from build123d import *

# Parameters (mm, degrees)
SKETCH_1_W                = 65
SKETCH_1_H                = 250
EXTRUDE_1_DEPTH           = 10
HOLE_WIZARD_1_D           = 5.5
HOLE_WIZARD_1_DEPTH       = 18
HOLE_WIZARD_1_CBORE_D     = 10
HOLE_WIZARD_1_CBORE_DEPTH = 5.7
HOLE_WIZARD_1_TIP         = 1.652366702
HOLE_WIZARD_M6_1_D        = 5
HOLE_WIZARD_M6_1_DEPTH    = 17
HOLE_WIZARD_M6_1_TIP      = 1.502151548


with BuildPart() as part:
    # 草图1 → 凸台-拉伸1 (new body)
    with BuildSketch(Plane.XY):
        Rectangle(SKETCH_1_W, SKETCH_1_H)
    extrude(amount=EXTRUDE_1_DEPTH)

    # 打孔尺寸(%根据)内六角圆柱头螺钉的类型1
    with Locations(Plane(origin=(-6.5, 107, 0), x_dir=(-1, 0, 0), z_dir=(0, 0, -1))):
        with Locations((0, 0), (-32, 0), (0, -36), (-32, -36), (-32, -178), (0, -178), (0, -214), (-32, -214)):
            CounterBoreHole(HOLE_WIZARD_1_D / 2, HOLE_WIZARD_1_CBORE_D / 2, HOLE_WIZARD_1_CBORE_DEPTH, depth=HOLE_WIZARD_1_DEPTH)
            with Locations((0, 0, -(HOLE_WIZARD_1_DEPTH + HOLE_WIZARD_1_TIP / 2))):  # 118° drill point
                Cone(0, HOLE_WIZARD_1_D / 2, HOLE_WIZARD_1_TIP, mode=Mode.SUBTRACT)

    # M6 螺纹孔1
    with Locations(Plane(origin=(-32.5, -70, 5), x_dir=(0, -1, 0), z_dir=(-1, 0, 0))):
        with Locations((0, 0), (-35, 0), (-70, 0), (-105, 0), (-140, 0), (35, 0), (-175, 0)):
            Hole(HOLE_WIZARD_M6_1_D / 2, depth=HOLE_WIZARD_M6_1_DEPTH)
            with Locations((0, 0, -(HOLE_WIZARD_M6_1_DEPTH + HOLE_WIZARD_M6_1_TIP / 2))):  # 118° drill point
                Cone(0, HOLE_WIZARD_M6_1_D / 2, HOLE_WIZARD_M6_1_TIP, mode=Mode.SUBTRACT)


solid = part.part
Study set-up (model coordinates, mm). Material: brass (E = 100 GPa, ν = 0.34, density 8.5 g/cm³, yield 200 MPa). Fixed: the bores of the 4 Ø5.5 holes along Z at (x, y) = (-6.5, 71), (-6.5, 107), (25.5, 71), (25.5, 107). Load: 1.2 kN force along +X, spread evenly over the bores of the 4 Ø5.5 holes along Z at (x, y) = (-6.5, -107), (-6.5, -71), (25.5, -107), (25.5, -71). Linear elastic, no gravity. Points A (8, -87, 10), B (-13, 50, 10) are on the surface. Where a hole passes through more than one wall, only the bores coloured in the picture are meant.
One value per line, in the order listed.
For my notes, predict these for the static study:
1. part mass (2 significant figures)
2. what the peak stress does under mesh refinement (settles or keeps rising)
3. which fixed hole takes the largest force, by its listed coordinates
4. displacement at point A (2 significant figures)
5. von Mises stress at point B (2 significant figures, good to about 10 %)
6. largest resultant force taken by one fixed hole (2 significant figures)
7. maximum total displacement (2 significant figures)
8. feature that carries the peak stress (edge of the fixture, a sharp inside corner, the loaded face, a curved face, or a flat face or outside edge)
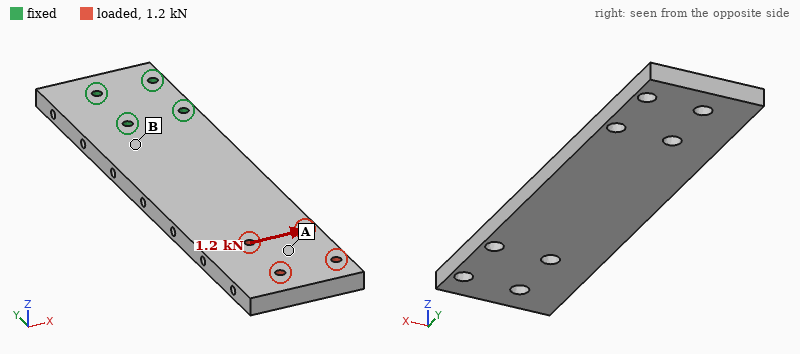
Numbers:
1.3 kg
keeps rising
(25.5, 71)
0.12 mm
14 MPa
3.6 kN
0.16 mm
edge of the fixture
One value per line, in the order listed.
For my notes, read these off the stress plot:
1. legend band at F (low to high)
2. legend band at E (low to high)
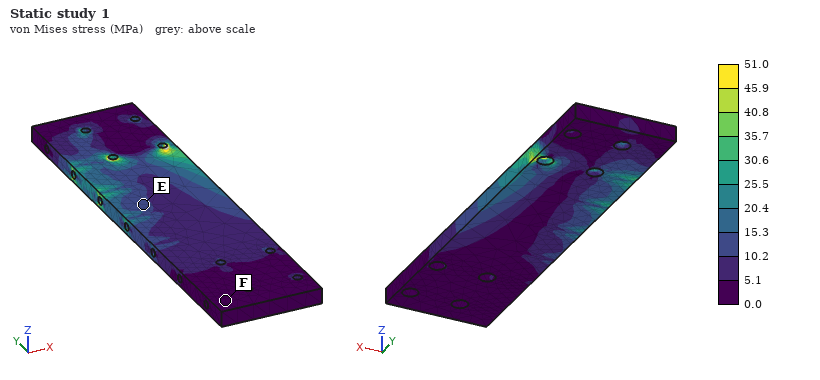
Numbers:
0.0 to 5.1 MPa
10.2 to 15.3 MPa
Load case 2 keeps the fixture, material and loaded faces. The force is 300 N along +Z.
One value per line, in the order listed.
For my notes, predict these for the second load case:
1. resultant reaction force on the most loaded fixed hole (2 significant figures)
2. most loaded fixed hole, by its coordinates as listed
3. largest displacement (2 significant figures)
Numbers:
1.6 kN
(-6.5, 71)
1.2 mm
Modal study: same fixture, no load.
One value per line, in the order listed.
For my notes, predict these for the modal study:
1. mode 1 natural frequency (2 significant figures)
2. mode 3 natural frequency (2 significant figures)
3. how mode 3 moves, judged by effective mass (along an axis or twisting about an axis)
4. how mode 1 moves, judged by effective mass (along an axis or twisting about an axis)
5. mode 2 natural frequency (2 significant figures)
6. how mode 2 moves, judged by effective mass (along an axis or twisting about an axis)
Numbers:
140 Hz
810 Hz
twisting about Y
along Z
730 Hz
along X
